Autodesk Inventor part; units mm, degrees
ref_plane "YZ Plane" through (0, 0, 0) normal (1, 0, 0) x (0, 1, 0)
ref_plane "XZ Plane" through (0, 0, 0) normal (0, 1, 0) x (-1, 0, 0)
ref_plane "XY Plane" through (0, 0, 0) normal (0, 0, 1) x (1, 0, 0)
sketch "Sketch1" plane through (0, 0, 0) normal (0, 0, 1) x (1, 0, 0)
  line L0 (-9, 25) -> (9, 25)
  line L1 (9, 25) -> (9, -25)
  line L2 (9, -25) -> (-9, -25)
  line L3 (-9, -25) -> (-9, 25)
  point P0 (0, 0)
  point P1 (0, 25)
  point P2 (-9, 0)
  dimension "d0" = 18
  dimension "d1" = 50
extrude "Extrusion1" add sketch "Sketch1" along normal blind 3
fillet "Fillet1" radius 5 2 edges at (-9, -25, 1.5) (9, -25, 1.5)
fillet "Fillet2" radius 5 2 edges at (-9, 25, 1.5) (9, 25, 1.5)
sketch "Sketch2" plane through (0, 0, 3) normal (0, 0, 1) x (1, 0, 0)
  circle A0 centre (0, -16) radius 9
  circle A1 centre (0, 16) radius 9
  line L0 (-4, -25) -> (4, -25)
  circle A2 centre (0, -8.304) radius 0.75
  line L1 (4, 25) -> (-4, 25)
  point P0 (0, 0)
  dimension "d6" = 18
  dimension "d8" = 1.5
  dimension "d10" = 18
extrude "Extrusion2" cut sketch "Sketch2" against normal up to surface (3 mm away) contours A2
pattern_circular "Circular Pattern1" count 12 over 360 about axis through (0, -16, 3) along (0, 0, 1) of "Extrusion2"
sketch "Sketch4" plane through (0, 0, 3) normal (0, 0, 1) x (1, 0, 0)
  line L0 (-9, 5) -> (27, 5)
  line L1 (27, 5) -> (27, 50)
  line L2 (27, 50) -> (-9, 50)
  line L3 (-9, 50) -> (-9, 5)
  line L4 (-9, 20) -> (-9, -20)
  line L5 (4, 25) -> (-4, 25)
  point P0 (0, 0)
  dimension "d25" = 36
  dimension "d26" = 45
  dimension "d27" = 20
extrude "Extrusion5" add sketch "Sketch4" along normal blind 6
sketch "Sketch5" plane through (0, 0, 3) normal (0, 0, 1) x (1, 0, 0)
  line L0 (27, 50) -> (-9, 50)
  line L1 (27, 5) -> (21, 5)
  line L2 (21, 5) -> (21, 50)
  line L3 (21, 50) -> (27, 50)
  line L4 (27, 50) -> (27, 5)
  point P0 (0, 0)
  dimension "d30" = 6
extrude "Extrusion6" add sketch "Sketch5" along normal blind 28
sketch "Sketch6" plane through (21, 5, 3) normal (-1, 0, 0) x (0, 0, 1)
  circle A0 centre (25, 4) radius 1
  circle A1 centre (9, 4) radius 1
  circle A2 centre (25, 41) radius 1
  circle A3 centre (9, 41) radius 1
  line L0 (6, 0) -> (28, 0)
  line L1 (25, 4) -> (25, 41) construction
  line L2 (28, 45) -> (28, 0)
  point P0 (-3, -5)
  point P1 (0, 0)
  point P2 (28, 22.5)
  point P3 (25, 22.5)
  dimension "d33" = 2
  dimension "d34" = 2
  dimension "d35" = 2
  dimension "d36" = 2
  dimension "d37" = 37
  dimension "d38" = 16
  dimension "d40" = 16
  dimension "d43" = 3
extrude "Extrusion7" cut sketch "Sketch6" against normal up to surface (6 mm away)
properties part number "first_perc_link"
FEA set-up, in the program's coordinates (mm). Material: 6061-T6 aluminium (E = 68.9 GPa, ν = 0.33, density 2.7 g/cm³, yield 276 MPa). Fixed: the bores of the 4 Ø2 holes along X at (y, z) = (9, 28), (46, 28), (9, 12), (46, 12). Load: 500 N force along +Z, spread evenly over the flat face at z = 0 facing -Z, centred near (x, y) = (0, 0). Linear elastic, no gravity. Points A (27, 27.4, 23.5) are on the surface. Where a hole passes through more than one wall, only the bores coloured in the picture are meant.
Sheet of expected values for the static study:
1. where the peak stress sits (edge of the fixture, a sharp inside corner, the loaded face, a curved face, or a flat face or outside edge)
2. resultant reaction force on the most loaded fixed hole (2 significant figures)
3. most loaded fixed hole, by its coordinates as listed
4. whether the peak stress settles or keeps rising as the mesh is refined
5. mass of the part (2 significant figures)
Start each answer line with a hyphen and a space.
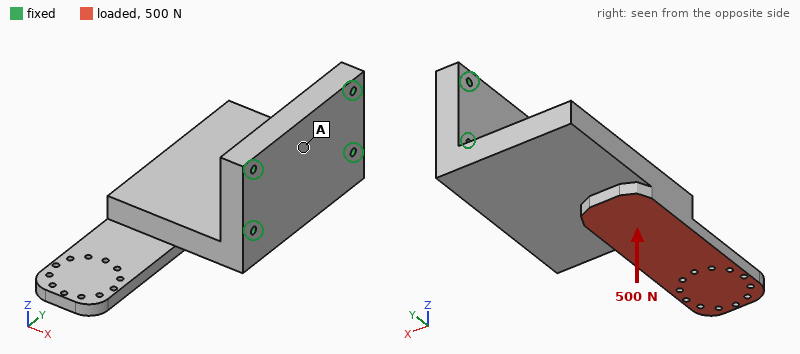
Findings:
- edge of the fixture
- 560 N
- (9, 12)
- keeps rising
- 49 g
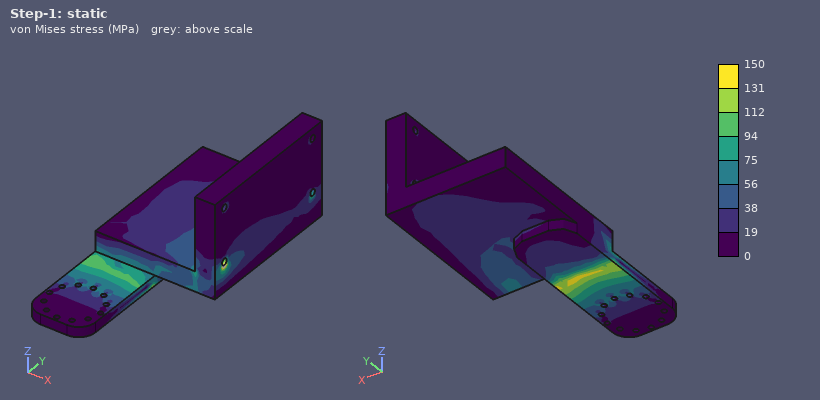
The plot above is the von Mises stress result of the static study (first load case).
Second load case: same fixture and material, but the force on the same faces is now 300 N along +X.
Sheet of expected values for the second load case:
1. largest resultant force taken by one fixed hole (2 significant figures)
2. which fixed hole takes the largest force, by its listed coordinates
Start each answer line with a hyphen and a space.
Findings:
- 430 N
- (9, 12)
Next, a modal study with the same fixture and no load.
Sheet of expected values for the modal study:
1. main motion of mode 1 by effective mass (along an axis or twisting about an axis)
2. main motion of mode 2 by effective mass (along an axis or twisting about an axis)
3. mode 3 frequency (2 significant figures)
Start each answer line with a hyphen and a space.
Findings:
- along Z
- along Z
- 6600 Hz
